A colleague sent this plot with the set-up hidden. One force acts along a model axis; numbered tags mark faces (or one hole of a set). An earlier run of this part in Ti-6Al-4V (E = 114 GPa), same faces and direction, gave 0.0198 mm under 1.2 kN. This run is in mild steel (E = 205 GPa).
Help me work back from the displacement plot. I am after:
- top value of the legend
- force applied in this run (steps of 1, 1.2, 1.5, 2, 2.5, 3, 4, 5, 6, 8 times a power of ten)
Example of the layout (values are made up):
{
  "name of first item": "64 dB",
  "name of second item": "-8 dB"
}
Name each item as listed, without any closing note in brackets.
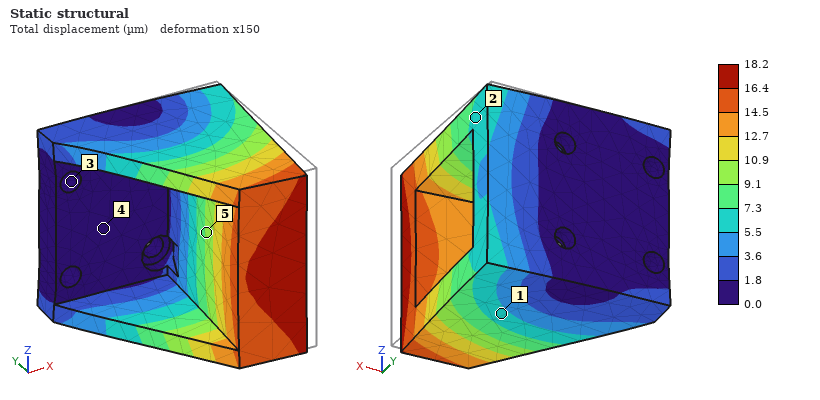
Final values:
{
  "top value of the legend": "18.2 µm",
  "force applied in this run": "2 kN"
}
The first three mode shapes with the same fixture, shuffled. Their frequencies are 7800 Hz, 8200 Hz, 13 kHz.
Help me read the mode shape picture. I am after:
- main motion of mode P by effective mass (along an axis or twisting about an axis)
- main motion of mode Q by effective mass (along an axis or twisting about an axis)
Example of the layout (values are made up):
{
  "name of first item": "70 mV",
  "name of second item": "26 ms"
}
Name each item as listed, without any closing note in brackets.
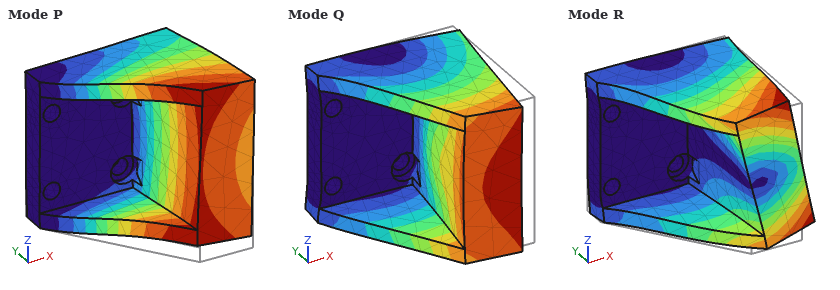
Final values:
{
  "main motion of mode P by effective mass": "along Z",
  "main motion of mode Q by effective mass": "along X"
}
